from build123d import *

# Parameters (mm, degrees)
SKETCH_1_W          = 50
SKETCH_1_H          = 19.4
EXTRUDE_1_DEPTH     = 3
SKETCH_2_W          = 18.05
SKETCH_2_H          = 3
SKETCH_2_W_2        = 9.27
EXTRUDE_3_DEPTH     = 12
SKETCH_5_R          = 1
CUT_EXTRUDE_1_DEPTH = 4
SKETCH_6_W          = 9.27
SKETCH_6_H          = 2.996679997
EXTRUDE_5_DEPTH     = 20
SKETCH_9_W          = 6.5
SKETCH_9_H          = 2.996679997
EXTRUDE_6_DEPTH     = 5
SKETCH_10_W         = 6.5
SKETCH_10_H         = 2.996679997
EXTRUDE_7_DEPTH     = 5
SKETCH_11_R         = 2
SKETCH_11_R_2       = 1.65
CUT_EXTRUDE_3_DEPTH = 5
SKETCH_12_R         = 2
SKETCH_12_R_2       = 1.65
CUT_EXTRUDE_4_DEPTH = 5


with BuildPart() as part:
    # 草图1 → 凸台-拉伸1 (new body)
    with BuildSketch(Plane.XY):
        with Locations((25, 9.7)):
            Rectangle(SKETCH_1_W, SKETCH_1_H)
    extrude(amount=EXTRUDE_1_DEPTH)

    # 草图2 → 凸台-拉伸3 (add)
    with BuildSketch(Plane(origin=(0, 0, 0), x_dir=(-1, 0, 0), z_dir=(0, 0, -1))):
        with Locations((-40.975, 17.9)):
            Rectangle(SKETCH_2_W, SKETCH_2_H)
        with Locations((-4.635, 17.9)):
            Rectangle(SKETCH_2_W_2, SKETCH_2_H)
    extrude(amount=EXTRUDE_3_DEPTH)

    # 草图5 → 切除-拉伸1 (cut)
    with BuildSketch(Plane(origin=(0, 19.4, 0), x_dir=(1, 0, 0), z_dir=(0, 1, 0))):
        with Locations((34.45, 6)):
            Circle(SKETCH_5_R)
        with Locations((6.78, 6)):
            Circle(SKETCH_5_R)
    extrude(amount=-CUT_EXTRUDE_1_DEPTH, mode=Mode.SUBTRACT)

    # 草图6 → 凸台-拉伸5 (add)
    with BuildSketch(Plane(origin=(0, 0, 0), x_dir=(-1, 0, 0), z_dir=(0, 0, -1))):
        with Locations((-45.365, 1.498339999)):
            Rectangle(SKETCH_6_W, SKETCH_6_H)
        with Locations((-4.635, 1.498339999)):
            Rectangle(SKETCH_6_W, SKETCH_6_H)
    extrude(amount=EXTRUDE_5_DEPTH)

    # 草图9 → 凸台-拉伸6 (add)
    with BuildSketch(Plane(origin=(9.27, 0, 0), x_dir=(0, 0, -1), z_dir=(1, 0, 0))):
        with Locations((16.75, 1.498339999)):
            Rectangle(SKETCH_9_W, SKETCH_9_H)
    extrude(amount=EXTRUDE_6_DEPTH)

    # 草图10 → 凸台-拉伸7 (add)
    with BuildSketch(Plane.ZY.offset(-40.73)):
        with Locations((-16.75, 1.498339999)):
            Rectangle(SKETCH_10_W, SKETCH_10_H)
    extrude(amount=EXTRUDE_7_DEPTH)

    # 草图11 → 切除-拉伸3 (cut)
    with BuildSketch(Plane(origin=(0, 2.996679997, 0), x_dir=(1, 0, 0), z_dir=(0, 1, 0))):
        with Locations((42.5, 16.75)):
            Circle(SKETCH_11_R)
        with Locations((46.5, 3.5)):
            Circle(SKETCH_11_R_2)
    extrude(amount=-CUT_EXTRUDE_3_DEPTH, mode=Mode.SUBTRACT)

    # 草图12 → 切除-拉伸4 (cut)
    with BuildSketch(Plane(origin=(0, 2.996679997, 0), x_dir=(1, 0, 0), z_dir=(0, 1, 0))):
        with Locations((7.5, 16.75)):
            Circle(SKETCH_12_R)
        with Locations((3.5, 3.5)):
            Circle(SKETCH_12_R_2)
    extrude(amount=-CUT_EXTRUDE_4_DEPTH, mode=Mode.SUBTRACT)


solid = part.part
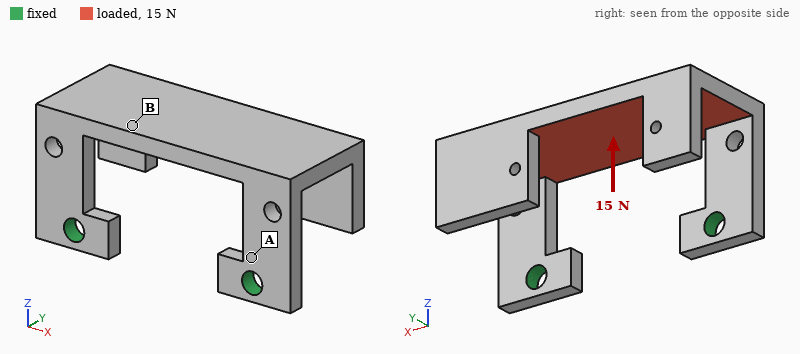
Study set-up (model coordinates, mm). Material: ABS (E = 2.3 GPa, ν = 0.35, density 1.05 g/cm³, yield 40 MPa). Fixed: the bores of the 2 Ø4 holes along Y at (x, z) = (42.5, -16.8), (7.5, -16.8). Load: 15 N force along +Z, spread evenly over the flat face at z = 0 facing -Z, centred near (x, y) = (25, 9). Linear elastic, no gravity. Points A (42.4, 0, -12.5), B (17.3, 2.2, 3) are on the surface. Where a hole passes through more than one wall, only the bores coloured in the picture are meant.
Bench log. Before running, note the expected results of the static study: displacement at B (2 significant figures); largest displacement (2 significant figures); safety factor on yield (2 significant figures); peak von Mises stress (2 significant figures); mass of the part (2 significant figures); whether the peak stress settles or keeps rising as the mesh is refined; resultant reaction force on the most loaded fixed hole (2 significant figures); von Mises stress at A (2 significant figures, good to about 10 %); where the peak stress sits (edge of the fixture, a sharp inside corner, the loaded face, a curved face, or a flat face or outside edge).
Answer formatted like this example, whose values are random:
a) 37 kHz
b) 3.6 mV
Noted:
a) 0.24 mm
b) 0.57 mm
c) 3.6
d) 11 MPa
e) 5.3 g
f) settles
g) 7.9 N
h) 4.6 MPa
i) a curved face
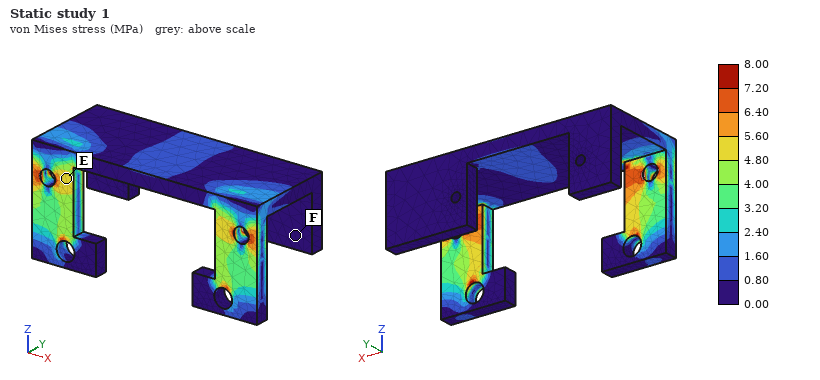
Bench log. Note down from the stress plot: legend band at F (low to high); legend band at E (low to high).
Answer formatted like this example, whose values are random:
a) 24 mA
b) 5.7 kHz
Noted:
a) 0.00 to 0.80 MPa
b) 4.80 to 5.60 MPa
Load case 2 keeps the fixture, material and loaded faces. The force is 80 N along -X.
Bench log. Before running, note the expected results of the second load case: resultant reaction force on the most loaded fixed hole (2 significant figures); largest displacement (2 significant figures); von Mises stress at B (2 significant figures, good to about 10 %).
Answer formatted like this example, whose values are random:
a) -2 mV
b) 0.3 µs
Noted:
a) 43 N
b) 0.62 mm
c) 2.2 MPa
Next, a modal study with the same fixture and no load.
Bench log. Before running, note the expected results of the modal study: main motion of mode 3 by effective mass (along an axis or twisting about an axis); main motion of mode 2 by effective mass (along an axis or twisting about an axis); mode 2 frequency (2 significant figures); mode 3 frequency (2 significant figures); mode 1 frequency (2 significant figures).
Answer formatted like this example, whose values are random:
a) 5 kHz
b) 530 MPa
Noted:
a) along Y
b) along X
c) 750 Hz
d) 970 Hz
e) 370 Hz
